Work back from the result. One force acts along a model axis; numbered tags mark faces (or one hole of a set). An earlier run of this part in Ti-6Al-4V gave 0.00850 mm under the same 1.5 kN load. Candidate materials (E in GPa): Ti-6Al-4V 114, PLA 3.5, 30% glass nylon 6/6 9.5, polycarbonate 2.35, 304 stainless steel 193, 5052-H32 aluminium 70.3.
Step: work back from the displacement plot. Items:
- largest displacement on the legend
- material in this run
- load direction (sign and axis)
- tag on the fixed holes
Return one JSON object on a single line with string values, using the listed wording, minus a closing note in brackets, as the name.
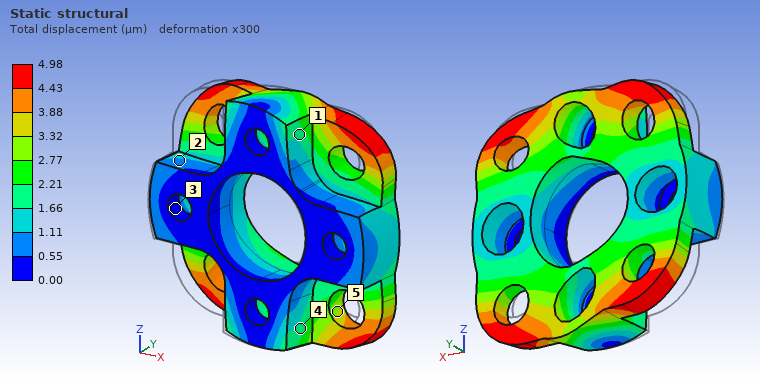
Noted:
{"largest displacement on the legend": "4.98 µm", "material in this run": "304 stainless steel", "load direction": "+X", "tag on the fixed holes": "3"}
